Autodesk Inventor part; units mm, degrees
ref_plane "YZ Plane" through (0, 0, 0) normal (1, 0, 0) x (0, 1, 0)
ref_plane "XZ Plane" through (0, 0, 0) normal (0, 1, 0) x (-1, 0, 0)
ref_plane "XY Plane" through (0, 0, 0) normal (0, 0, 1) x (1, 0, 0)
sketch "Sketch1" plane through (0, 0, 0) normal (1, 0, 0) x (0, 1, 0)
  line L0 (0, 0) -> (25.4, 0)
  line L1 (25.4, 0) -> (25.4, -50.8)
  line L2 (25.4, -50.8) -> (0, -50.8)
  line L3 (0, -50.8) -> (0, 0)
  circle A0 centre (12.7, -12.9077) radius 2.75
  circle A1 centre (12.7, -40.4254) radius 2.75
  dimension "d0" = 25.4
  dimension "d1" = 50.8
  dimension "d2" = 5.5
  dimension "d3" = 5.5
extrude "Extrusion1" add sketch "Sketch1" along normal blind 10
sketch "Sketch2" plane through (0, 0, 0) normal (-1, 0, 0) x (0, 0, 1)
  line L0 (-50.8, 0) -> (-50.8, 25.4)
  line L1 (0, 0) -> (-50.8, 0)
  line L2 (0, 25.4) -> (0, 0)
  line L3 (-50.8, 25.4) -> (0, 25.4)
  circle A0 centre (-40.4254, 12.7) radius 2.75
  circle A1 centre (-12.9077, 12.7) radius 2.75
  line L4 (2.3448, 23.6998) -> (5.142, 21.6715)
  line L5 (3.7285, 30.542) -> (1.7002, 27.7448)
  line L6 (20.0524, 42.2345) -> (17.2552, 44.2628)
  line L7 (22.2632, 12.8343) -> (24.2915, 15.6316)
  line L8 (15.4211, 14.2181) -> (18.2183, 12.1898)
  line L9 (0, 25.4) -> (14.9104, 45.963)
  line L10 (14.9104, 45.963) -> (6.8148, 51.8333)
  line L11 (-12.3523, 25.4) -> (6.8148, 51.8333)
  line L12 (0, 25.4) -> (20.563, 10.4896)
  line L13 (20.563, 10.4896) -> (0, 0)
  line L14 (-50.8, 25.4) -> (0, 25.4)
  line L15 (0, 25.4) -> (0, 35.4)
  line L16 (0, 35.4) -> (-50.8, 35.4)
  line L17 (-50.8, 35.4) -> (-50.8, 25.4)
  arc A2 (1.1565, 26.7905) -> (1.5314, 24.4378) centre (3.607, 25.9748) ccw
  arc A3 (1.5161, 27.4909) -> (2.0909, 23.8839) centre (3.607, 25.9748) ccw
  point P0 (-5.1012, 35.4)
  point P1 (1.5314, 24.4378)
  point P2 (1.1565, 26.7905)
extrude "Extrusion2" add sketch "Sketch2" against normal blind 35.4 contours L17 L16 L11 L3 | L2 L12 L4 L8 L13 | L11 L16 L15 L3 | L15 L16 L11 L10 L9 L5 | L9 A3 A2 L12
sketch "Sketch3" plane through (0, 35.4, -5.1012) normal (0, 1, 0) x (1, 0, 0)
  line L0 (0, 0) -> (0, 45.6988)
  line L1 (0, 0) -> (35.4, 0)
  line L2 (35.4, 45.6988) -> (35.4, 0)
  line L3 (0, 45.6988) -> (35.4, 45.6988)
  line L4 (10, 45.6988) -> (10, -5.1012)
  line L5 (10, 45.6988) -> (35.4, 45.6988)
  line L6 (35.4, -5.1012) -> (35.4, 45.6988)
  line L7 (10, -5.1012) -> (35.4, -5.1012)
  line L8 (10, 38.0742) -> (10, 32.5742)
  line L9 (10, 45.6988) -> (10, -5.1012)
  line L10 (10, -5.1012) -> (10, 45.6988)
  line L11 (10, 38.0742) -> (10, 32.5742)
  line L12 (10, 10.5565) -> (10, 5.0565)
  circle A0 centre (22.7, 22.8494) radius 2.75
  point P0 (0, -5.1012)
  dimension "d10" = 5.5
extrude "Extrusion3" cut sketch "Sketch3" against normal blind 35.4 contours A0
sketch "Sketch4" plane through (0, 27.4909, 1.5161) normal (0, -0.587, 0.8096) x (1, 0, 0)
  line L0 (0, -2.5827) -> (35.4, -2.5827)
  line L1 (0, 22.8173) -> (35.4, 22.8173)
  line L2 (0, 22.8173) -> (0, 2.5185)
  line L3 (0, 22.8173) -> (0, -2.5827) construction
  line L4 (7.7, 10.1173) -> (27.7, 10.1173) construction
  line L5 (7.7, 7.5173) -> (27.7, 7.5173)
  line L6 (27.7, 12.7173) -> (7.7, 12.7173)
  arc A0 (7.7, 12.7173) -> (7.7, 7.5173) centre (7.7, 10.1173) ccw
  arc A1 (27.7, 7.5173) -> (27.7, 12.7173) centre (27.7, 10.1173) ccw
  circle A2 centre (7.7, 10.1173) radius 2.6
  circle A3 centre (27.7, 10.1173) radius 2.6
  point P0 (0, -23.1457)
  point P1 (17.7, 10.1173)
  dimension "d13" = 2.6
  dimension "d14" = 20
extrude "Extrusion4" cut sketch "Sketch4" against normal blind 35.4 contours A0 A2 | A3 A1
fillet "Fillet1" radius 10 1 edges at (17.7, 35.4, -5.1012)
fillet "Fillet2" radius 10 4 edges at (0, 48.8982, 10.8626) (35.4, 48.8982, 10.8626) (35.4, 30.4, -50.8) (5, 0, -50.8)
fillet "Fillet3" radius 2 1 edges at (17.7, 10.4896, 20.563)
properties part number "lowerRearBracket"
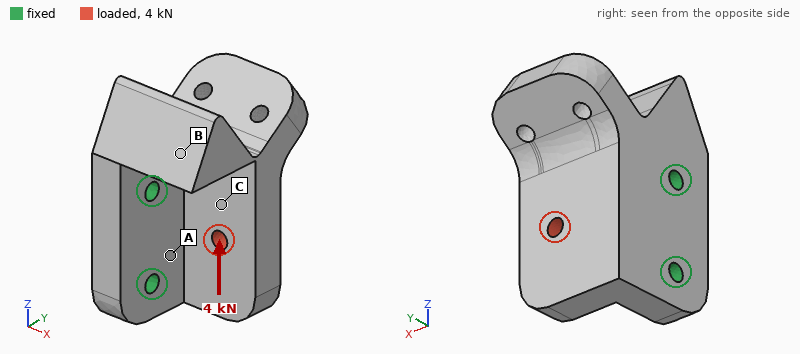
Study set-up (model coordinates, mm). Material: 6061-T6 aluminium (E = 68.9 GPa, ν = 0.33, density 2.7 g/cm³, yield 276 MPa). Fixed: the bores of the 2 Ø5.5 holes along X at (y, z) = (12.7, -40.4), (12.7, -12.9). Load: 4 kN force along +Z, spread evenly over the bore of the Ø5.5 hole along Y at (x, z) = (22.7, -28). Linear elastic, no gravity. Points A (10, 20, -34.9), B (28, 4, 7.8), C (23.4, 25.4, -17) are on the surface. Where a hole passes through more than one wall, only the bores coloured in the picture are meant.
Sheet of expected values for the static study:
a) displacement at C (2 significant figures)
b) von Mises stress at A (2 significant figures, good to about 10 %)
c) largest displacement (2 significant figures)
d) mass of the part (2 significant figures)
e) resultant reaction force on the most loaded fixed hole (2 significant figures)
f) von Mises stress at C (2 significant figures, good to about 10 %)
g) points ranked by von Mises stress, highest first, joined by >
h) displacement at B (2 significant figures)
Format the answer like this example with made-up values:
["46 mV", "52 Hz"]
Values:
["31 µm", "44 MPa", "62 µm", "120 g", "3.6 kN", "22 MPa", "A > C > B", "24 µm"]
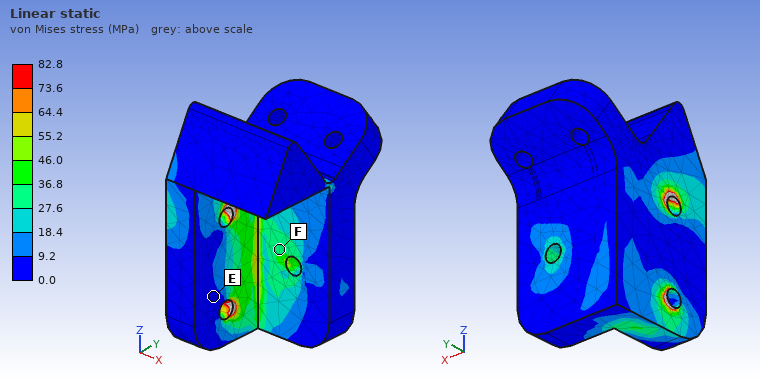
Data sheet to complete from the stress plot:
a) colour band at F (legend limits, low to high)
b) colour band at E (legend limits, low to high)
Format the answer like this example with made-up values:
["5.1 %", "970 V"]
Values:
["27.6 to 36.8 MPa", "0.0 to 9.2 MPa"]
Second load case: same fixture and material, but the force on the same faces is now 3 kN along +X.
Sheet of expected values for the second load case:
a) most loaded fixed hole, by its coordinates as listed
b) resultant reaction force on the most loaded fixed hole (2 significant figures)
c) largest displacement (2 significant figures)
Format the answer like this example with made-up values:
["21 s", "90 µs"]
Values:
["(12.7, -40.4)", "1.6 kN", "60 µm"]
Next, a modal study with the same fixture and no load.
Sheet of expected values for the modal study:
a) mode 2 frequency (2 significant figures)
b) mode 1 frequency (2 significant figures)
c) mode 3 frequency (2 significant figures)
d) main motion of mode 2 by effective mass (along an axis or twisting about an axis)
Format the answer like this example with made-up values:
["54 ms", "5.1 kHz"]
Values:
["5300 Hz", "3400 Hz", "7000 Hz", "along Z"]
